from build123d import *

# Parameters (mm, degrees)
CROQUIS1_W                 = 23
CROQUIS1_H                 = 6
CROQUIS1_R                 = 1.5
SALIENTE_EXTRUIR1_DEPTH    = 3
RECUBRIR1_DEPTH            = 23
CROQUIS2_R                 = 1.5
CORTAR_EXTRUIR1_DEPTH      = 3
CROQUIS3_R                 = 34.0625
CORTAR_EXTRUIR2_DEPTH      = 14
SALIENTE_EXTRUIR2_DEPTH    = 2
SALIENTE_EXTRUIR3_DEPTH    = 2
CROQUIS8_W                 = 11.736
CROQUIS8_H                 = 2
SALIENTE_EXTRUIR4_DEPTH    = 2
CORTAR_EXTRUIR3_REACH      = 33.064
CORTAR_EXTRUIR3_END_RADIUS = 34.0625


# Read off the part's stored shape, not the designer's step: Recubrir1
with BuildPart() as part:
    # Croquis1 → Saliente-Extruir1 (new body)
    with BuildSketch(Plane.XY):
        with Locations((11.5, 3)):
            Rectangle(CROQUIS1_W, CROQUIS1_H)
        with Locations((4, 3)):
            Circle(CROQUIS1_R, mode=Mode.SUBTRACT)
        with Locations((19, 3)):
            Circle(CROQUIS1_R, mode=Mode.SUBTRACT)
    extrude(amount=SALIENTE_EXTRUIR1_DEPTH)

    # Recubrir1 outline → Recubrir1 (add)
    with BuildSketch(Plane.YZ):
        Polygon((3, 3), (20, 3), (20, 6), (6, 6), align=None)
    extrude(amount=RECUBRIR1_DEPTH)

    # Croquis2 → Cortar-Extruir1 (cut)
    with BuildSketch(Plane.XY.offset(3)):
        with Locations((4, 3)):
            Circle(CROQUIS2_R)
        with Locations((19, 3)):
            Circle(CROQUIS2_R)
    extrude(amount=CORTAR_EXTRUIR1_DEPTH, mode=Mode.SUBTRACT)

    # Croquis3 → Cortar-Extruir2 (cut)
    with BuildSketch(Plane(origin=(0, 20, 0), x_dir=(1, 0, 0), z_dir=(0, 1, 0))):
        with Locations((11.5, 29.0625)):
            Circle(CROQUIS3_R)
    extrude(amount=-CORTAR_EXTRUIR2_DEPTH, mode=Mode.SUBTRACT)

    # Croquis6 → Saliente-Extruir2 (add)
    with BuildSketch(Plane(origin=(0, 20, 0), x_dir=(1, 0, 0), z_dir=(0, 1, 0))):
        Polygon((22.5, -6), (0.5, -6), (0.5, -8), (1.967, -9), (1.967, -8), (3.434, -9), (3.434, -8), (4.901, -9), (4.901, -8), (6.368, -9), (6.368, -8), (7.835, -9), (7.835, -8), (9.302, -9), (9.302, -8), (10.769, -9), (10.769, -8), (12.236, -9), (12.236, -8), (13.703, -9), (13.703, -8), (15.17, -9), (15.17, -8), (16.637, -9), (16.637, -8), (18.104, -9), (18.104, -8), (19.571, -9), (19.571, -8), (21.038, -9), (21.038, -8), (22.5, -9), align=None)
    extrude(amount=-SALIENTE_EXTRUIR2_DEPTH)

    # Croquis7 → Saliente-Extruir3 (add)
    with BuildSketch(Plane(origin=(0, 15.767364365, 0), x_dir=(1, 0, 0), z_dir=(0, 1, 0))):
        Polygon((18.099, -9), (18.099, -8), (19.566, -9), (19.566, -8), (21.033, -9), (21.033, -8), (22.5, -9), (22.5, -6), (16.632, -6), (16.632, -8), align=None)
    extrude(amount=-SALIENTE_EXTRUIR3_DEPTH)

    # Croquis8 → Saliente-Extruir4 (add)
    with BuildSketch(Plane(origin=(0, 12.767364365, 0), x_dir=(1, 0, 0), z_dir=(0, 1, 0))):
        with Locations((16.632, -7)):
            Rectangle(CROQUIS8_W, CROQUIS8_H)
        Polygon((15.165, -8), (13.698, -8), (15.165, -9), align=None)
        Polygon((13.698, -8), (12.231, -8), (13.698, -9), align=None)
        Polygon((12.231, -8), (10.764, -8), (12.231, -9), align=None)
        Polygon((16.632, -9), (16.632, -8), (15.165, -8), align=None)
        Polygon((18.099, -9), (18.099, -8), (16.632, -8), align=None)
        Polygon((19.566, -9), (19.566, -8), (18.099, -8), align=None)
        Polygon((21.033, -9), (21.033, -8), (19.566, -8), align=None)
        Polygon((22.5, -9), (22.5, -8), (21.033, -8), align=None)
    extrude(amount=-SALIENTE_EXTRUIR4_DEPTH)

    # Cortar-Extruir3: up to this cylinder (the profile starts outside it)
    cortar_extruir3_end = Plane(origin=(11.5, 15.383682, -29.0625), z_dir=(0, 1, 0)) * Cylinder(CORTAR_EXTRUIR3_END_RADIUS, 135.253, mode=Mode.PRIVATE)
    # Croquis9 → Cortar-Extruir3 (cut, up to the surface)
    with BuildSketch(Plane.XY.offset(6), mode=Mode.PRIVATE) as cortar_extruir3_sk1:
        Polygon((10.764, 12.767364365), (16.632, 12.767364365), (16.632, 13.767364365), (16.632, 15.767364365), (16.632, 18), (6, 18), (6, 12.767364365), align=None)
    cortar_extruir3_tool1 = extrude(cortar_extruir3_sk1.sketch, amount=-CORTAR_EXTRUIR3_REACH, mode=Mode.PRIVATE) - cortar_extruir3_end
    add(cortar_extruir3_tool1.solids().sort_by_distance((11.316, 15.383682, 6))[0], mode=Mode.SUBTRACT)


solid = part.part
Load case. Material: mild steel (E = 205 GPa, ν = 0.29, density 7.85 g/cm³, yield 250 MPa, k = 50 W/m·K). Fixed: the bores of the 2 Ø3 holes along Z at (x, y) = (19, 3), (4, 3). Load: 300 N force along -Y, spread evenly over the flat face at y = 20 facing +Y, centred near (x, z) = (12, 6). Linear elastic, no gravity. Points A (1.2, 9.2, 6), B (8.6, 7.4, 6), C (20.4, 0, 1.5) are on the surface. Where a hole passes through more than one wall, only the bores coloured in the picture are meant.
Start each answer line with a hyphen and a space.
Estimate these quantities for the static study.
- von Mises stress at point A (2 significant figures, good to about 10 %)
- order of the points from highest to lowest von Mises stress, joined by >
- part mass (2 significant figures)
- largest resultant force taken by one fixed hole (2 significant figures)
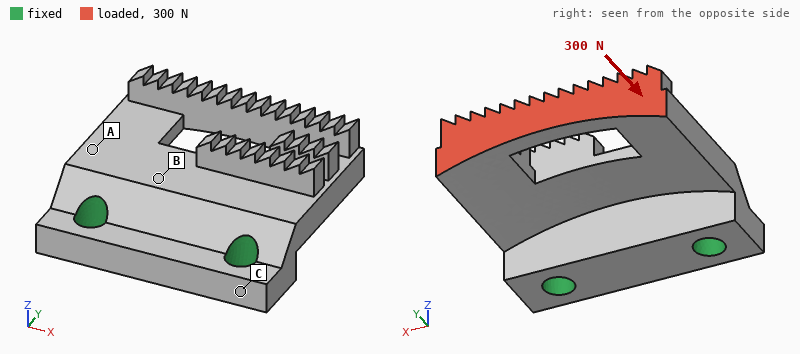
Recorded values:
- 41 MPa
- A > B > C
- 8.9 g
- 150 N
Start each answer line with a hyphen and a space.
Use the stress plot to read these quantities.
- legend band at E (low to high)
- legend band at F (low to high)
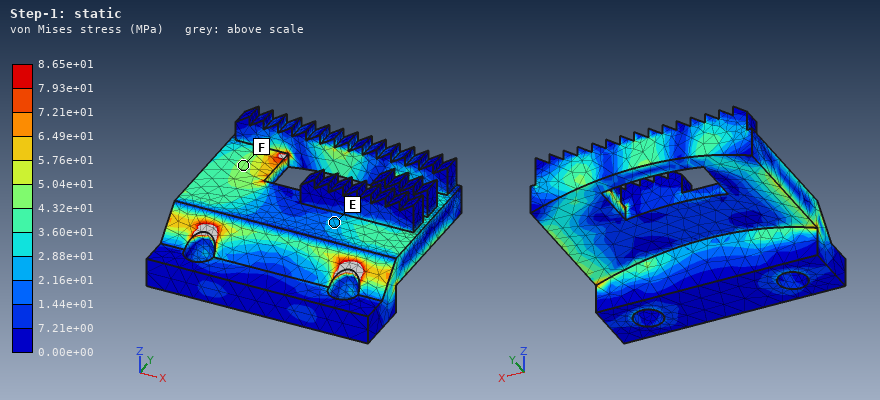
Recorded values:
- 2.16e+01 to 2.88e+01 MPa
- 4.32e+01 to 5.04e+01 MPa
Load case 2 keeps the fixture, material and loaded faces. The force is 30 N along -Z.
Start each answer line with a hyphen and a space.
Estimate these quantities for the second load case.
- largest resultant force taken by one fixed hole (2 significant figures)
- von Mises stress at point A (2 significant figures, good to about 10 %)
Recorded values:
- 15 N
- 26 MPa
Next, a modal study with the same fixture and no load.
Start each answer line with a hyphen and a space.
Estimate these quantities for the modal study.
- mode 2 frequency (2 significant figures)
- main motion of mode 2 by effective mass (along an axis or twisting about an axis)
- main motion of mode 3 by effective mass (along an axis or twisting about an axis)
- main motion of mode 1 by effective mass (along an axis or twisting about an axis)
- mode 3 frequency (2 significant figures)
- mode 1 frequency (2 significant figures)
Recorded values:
- 8400 Hz
- twisting about Y
- along X
- along Z
- 19 kHz
- 4700 Hz
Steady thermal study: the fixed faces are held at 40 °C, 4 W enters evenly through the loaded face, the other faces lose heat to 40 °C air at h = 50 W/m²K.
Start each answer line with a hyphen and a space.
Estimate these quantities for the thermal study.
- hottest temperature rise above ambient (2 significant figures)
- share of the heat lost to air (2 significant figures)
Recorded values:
- 44 K
- 24 %
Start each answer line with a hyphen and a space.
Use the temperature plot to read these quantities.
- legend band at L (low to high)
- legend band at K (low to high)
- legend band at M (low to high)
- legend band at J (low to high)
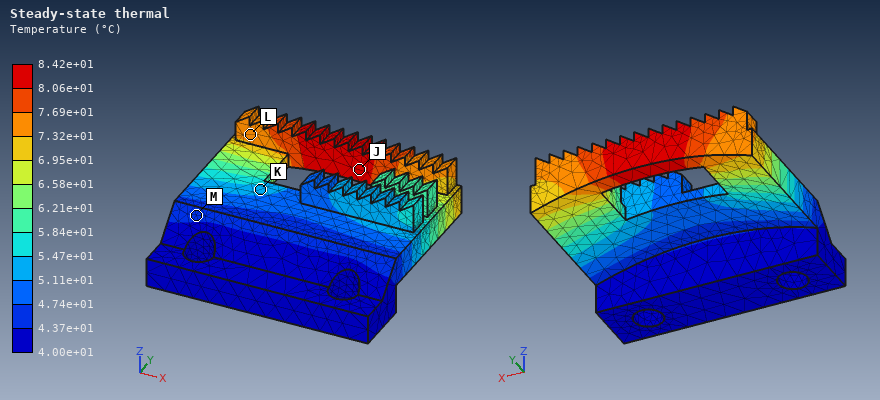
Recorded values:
- 7.32e+01 to 7.69e+01 °C
- 5.11e+01 to 5.47e+01 °C
- 4.37e+01 to 4.74e+01 °C
- 8.06e+01 to 8.42e+01 °C
